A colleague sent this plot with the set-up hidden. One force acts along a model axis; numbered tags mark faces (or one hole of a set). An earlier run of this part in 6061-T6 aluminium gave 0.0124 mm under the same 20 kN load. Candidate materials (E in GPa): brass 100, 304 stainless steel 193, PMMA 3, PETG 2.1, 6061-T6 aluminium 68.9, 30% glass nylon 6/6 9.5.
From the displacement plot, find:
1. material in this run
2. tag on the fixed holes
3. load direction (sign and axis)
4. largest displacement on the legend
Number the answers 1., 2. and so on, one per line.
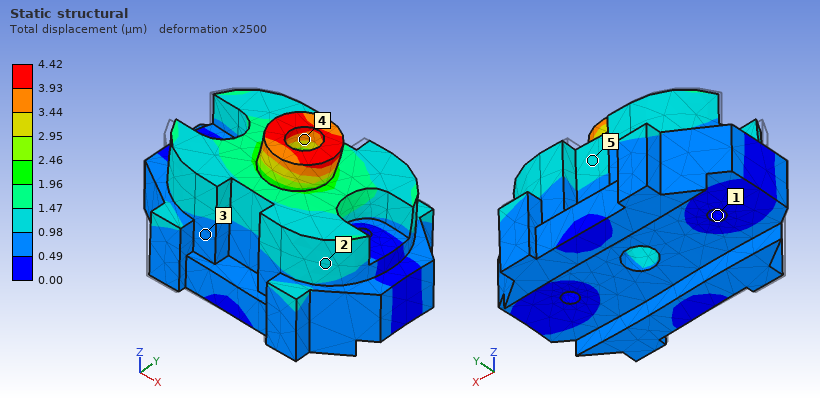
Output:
1. 304 stainless steel
2. 1
3. +X
4. 4.42 µm
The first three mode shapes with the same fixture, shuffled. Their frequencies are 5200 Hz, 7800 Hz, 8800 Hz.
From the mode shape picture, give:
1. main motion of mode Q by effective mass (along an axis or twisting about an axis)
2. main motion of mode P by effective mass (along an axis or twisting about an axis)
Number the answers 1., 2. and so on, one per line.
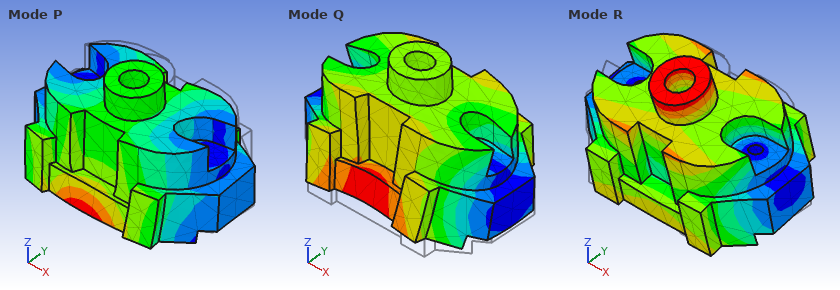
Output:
1. along Z
2. along Y
